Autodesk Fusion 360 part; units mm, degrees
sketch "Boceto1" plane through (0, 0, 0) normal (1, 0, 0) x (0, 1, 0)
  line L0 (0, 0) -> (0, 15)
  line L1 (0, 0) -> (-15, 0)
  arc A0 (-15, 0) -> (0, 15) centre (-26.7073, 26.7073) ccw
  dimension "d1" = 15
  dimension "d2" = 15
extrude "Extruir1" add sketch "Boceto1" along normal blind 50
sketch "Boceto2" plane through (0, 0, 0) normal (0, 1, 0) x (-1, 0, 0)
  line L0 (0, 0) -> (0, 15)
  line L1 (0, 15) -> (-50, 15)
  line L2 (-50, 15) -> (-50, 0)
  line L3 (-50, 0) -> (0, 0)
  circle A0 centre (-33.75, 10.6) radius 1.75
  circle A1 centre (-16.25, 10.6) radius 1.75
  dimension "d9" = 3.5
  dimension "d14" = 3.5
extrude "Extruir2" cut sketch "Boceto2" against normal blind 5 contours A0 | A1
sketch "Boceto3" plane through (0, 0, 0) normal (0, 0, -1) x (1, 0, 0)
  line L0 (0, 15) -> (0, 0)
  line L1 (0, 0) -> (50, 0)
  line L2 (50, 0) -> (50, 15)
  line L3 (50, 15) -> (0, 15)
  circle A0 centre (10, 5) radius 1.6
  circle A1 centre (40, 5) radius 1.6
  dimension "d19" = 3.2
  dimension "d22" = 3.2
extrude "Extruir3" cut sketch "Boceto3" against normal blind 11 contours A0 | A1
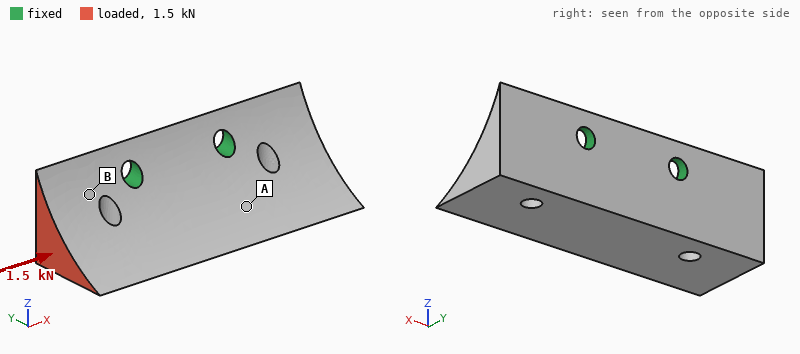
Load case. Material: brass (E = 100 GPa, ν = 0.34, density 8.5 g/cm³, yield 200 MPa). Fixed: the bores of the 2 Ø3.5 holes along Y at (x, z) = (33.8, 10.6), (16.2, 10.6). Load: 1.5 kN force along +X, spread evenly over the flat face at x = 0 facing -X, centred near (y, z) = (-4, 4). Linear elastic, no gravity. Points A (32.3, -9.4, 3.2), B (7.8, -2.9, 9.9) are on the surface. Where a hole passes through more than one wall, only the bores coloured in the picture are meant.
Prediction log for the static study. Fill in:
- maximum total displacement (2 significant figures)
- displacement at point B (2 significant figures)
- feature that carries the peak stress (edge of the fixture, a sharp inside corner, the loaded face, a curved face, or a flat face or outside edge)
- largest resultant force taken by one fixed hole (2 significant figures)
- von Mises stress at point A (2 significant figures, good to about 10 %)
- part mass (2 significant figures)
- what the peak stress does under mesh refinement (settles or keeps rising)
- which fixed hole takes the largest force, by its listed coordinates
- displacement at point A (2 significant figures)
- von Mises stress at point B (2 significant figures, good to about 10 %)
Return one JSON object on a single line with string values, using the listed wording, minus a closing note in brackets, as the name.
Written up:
{"maximum total displacement": "12 µm", "displacement at point B": "4.1 µm", "feature that carries the peak stress": "edge of the fixture", "largest resultant force taken by one fixed hole": "1.1 kN", "von Mises stress at point A": "8.8 MPa", "part mass": "34 g", "what the peak stress does under mesh refinement": "keeps rising", "which fixed hole takes the largest force, by its listed coordinates": "(16.2, 10.6)", "displacement at point A": "3.5 µm", "von Mises stress at point B": "23 MPa"}
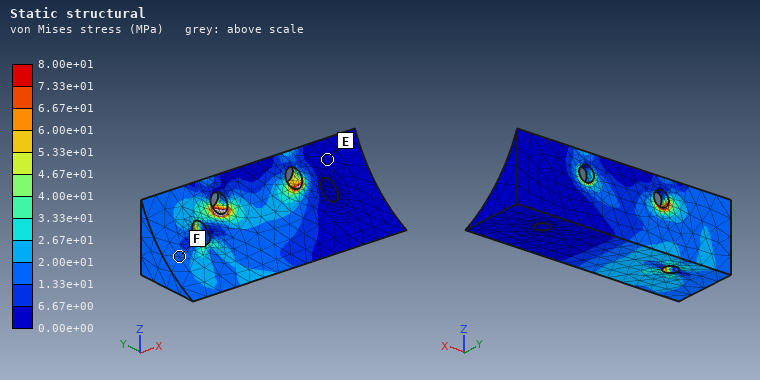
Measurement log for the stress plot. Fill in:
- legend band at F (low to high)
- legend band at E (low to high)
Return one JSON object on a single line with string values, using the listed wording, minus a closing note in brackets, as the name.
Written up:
{"legend band at F": "1.33e+01 to 2.00e+01 MPa", "legend band at E": "0.00e+00 to 6.67e+00 MPa"}
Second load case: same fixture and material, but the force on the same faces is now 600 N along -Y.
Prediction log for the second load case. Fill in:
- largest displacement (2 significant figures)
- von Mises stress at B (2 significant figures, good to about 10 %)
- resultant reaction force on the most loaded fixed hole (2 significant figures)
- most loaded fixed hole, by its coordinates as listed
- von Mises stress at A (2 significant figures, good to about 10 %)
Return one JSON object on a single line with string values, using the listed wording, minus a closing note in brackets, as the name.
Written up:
{"largest displacement": "82 µm", "von Mises stress at B": "26 MPa", "resultant reaction force on the most loaded fixed hole": "1.0 kN", "most loaded fixed hole, by its coordinates as listed": "(16.2, 10.6)", "von Mises stress at A": "27 MPa"}
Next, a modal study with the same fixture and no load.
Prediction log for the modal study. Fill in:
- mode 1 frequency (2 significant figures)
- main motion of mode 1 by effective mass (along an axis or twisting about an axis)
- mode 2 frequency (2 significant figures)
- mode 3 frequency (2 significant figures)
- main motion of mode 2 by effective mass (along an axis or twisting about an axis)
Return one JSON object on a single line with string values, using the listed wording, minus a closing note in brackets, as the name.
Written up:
{"mode 1 frequency": "5700 Hz", "main motion of mode 1 by effective mass": "along Y", "mode 2 frequency": "6300 Hz", "mode 3 frequency": "11 kHz", "main motion of mode 2 by effective mass": "twisting about Z"}
